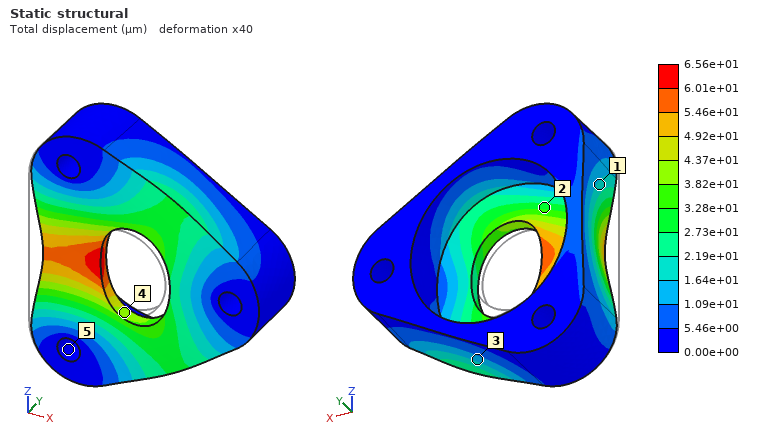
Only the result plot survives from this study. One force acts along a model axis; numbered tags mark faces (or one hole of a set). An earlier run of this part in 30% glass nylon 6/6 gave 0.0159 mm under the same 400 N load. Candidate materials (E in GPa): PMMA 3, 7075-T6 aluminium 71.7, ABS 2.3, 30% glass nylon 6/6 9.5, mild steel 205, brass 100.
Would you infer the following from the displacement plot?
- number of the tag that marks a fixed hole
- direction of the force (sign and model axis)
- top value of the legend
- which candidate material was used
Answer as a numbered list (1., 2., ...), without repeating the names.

1. 5
2. +X
3. 6.56e+01 µm
4. ABS
